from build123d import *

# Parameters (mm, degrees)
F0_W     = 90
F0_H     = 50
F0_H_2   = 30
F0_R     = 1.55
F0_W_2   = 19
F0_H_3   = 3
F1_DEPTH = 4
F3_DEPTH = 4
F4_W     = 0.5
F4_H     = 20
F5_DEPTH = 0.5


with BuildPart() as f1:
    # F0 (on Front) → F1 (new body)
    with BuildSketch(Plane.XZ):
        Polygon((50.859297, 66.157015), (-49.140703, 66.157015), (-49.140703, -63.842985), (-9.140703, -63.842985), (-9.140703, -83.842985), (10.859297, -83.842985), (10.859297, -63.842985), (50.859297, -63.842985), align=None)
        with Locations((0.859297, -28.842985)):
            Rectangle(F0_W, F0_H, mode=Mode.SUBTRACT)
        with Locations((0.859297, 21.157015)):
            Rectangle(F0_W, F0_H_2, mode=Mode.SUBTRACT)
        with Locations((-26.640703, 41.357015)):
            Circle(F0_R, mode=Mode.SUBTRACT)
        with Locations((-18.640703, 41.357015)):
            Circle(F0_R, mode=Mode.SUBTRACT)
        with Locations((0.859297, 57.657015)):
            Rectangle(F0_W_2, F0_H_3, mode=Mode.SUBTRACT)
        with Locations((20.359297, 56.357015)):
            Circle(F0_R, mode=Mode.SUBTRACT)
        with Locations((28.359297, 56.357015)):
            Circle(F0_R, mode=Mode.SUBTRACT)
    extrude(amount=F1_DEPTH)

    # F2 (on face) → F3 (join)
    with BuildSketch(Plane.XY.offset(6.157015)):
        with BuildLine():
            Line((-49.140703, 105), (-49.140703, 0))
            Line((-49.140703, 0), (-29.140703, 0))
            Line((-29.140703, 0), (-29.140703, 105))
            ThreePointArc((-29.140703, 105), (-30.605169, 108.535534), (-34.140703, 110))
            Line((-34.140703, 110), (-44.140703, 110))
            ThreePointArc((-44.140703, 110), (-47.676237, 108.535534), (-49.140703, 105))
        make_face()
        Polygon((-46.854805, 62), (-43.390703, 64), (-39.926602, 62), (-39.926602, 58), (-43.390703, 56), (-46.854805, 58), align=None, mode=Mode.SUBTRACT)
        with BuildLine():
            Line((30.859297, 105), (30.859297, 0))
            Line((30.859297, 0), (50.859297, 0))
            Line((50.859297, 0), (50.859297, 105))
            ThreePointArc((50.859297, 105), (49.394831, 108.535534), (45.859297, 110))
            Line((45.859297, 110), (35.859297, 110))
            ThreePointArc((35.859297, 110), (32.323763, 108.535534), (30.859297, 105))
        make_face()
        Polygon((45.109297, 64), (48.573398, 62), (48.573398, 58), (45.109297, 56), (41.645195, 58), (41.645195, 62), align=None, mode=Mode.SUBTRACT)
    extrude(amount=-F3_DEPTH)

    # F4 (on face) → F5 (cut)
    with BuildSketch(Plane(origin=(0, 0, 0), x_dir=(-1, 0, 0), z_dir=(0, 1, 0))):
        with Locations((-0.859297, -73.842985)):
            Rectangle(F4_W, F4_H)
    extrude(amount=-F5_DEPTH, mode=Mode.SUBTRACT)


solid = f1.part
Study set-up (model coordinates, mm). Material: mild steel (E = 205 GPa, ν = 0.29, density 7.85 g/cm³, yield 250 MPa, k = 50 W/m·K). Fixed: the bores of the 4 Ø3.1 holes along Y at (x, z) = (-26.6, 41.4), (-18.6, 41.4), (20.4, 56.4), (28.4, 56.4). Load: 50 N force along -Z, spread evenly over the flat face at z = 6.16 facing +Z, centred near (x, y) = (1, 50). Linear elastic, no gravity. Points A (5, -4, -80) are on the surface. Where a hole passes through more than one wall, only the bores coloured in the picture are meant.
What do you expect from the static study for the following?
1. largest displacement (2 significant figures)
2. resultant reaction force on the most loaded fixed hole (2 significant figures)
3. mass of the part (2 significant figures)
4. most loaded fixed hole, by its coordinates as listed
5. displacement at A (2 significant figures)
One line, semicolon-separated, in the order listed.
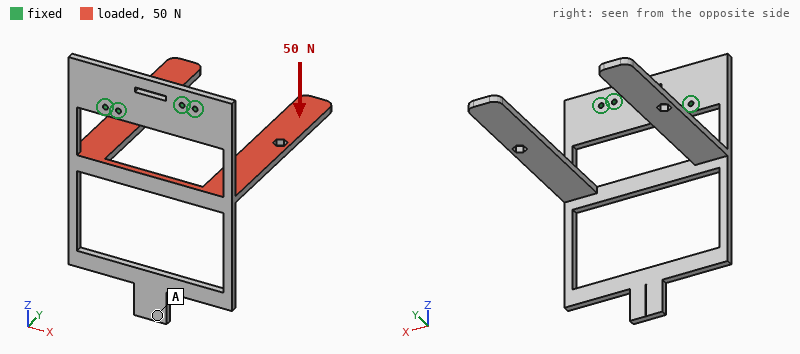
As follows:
1.3 mm; 44 N; 330 g; (28.4, 56.4); 0.98 mm
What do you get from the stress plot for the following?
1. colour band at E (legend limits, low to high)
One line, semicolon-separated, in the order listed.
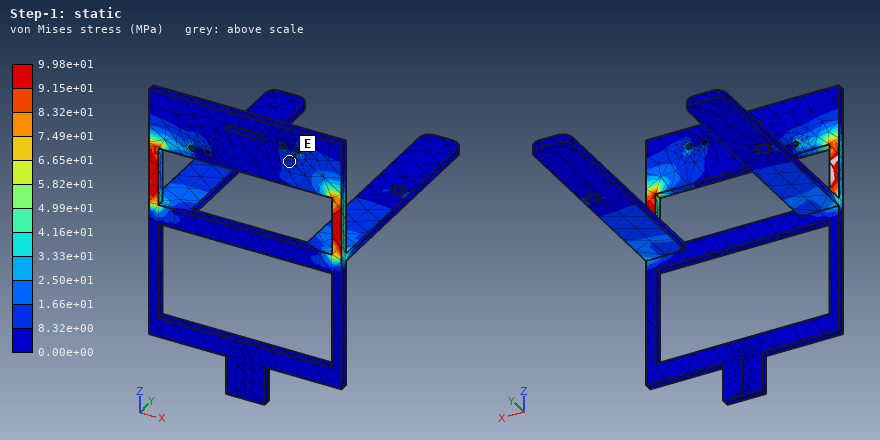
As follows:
8.32e+00 to 1.66e+01 MPa
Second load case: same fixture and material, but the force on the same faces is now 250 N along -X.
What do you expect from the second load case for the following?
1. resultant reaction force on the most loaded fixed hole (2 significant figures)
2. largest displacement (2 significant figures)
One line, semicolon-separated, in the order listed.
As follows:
360 N; 1.2 mm
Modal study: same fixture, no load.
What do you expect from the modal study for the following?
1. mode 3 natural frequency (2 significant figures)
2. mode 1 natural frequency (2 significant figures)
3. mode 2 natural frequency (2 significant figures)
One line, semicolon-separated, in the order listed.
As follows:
210 Hz; 79 Hz; 170 Hz
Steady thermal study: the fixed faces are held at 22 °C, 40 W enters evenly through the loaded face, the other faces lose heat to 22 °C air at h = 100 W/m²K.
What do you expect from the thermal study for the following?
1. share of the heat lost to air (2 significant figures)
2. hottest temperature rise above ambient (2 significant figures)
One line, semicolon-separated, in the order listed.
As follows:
99 %; 54 K
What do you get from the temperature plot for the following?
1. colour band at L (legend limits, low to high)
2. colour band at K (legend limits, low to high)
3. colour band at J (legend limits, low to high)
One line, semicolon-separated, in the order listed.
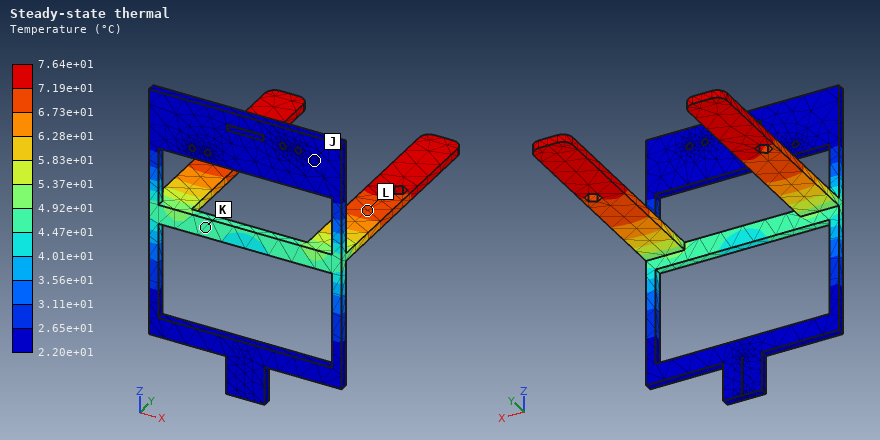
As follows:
6.73e+01 to 7.19e+01 °C; 4.47e+01 to 4.92e+01 °C; 2.20e+01 to 2.65e+01 °C
